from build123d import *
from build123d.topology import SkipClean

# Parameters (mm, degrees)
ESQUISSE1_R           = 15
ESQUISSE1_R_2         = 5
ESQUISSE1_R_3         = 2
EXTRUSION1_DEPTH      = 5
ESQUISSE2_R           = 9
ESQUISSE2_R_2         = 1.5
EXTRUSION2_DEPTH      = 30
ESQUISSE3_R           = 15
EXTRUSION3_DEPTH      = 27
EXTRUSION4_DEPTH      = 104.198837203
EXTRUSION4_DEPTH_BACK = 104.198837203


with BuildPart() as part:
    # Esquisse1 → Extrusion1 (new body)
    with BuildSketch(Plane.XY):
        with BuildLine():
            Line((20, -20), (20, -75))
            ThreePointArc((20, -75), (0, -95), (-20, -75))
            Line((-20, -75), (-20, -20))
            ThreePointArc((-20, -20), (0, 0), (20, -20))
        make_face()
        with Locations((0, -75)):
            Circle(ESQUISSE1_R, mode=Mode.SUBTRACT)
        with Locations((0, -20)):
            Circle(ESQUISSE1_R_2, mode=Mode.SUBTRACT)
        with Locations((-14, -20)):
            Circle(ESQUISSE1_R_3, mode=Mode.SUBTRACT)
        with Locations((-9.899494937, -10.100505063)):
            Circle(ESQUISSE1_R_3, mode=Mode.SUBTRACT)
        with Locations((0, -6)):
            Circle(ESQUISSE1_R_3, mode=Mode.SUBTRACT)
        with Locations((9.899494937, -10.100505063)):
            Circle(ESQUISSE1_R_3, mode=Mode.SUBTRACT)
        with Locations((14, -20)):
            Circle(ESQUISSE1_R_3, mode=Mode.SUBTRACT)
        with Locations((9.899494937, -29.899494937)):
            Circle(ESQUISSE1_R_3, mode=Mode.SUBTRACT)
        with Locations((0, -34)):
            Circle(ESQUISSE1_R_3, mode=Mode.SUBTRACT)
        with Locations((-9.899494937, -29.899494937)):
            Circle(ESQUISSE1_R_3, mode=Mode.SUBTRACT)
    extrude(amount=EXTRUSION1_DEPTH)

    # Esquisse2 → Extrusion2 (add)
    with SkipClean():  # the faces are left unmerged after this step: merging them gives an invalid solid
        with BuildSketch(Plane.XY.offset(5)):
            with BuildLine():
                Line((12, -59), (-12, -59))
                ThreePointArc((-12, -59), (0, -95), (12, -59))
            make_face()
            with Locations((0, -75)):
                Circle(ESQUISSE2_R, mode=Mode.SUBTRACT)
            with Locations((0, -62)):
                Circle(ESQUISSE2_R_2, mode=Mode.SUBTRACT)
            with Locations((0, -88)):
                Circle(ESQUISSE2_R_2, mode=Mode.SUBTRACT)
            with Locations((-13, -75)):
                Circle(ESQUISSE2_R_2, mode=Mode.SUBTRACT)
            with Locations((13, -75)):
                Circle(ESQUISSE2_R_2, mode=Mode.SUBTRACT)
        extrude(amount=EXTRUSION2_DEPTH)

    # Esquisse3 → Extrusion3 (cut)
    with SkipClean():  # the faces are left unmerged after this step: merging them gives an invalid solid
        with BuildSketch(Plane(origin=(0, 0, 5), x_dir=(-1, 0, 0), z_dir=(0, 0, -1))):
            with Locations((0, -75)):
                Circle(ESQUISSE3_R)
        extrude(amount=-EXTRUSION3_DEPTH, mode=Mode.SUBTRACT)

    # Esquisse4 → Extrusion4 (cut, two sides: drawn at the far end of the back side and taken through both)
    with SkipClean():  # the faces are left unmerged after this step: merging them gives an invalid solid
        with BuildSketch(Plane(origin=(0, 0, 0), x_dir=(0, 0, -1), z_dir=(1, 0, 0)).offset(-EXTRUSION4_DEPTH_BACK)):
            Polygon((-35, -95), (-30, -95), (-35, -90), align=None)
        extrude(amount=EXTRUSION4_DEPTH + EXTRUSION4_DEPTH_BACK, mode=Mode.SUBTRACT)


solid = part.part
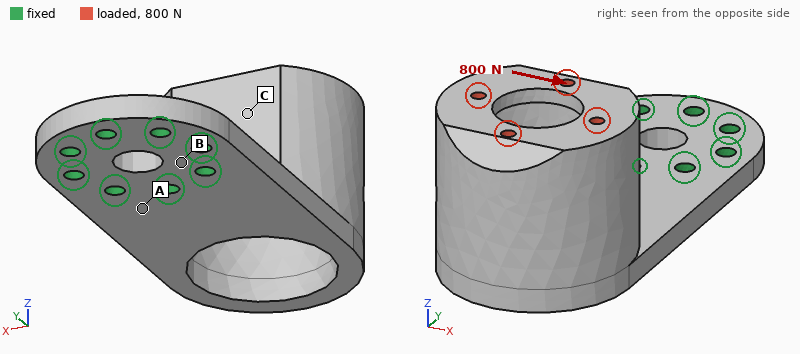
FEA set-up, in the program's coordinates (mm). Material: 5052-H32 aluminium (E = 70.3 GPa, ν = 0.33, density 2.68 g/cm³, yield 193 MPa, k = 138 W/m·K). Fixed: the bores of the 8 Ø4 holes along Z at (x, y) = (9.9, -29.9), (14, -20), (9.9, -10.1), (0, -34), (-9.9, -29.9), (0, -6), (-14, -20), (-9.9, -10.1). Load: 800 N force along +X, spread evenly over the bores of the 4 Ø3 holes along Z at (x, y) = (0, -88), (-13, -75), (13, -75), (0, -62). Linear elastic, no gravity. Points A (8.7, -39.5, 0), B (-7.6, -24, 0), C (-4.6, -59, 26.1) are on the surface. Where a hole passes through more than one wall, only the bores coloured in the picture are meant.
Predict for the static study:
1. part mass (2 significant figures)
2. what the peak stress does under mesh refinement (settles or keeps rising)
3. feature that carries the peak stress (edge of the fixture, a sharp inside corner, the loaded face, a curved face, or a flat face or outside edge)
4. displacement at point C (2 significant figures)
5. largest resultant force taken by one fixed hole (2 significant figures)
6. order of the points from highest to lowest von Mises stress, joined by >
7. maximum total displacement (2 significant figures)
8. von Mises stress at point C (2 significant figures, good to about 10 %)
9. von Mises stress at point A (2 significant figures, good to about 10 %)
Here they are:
76 g
keeps rising
edge of the fixture
0.29 mm
1.2 kN
A > C > B
0.46 mm
29 MPa
82 MPa
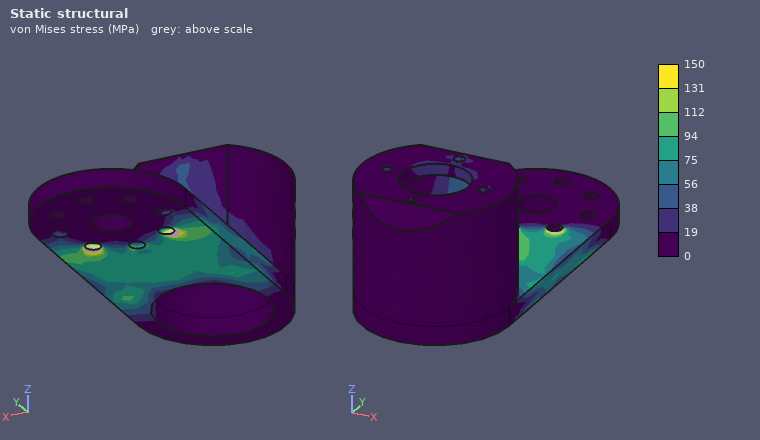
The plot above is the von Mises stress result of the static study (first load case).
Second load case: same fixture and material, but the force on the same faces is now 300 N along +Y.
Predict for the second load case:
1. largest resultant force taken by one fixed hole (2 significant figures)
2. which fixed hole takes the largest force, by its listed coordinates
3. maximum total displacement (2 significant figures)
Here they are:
390 N
(0, -34)
0.55 mm
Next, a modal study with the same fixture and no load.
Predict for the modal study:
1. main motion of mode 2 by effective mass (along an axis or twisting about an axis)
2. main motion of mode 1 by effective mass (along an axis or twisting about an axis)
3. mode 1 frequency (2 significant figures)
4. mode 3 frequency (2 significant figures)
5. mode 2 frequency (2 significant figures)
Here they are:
along X
along Z
600 Hz
3500 Hz
1400 Hz
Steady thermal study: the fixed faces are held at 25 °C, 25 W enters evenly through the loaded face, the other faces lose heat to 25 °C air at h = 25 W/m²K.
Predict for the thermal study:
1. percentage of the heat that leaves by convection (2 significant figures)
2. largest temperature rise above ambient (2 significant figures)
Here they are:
31 %
41 K
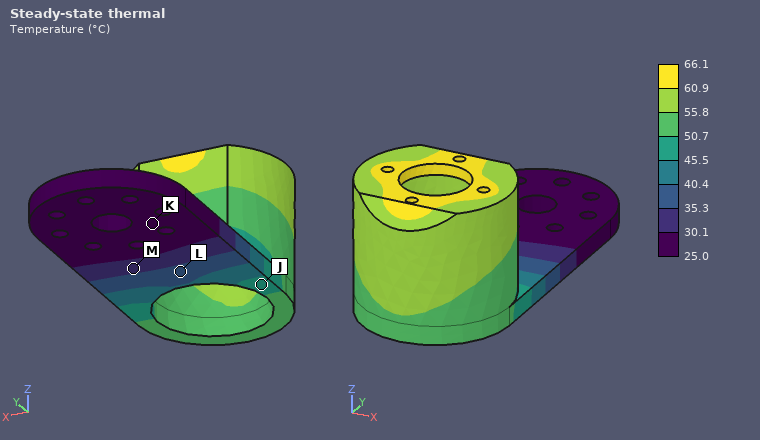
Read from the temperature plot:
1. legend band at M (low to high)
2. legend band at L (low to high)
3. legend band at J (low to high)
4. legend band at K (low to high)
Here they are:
30.1 to 35.3 °C
35.3 to 40.4 °C
45.5 to 50.7 °C
25.0 to 30.1 °C
